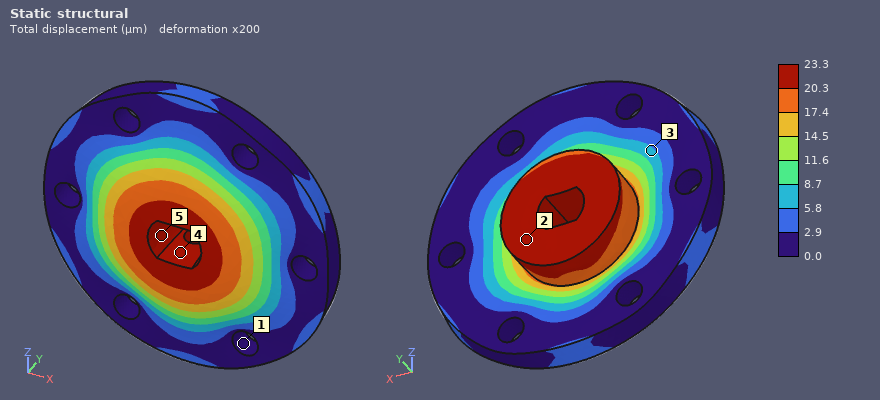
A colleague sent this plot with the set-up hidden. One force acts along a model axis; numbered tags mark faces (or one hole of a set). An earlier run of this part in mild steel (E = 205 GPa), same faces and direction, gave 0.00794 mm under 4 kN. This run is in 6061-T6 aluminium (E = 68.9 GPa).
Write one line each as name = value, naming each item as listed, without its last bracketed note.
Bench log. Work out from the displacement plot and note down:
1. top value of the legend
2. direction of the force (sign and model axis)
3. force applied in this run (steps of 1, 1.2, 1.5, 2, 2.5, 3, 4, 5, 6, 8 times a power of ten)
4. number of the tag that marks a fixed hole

top value of the legend = 23.3 µm
direction of the force = -Y
force applied in this run = 4 kN
number of the tag that marks a fixed hole = 1
